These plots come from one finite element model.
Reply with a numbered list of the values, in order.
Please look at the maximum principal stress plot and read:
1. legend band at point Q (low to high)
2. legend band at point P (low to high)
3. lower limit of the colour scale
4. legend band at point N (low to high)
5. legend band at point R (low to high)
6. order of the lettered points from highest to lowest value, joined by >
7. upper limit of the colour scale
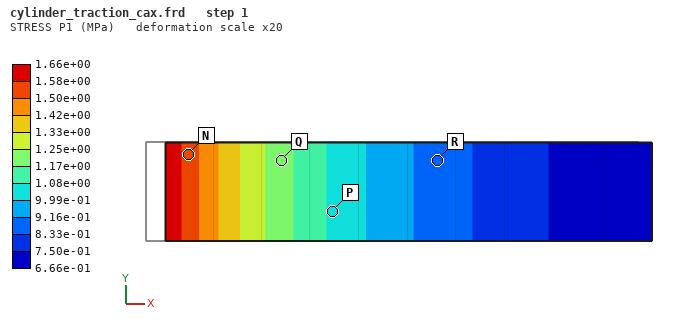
1. 1.17e+00 to 1.25e+00 MPa
2. 9.99e-01 to 1.08e+00 MPa
3. 6.66e-01 MPa
4. 1.50e+00 to 1.58e+00 MPa
5. 8.33e-01 to 9.16e-01 MPa
6. N > Q > P > R
7. 1.66e+00 MPa
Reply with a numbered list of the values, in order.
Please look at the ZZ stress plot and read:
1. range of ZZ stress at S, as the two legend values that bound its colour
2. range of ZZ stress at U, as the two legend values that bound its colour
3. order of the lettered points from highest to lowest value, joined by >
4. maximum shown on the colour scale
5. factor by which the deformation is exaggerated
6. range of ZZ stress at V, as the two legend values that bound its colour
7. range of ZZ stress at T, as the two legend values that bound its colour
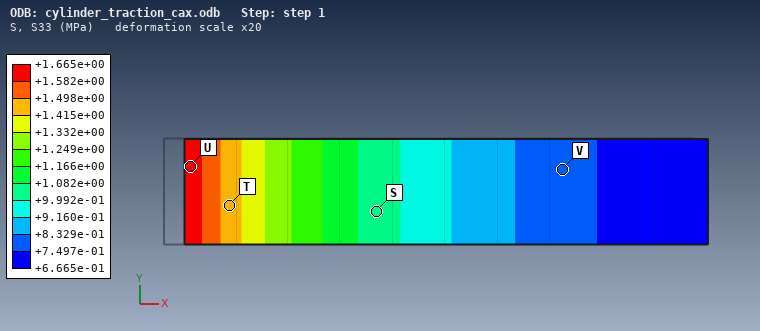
1. +9.992e-01 to +1.082e+00 MPa
2. +1.582e+00 to +1.665e+00 MPa
3. U > T > S > V
4. +1.665e+00 MPa
5. 20
6. +7.497e-01 to +8.329e-01 MPa
7. +1.415e+00 to +1.498e+00 MPa
